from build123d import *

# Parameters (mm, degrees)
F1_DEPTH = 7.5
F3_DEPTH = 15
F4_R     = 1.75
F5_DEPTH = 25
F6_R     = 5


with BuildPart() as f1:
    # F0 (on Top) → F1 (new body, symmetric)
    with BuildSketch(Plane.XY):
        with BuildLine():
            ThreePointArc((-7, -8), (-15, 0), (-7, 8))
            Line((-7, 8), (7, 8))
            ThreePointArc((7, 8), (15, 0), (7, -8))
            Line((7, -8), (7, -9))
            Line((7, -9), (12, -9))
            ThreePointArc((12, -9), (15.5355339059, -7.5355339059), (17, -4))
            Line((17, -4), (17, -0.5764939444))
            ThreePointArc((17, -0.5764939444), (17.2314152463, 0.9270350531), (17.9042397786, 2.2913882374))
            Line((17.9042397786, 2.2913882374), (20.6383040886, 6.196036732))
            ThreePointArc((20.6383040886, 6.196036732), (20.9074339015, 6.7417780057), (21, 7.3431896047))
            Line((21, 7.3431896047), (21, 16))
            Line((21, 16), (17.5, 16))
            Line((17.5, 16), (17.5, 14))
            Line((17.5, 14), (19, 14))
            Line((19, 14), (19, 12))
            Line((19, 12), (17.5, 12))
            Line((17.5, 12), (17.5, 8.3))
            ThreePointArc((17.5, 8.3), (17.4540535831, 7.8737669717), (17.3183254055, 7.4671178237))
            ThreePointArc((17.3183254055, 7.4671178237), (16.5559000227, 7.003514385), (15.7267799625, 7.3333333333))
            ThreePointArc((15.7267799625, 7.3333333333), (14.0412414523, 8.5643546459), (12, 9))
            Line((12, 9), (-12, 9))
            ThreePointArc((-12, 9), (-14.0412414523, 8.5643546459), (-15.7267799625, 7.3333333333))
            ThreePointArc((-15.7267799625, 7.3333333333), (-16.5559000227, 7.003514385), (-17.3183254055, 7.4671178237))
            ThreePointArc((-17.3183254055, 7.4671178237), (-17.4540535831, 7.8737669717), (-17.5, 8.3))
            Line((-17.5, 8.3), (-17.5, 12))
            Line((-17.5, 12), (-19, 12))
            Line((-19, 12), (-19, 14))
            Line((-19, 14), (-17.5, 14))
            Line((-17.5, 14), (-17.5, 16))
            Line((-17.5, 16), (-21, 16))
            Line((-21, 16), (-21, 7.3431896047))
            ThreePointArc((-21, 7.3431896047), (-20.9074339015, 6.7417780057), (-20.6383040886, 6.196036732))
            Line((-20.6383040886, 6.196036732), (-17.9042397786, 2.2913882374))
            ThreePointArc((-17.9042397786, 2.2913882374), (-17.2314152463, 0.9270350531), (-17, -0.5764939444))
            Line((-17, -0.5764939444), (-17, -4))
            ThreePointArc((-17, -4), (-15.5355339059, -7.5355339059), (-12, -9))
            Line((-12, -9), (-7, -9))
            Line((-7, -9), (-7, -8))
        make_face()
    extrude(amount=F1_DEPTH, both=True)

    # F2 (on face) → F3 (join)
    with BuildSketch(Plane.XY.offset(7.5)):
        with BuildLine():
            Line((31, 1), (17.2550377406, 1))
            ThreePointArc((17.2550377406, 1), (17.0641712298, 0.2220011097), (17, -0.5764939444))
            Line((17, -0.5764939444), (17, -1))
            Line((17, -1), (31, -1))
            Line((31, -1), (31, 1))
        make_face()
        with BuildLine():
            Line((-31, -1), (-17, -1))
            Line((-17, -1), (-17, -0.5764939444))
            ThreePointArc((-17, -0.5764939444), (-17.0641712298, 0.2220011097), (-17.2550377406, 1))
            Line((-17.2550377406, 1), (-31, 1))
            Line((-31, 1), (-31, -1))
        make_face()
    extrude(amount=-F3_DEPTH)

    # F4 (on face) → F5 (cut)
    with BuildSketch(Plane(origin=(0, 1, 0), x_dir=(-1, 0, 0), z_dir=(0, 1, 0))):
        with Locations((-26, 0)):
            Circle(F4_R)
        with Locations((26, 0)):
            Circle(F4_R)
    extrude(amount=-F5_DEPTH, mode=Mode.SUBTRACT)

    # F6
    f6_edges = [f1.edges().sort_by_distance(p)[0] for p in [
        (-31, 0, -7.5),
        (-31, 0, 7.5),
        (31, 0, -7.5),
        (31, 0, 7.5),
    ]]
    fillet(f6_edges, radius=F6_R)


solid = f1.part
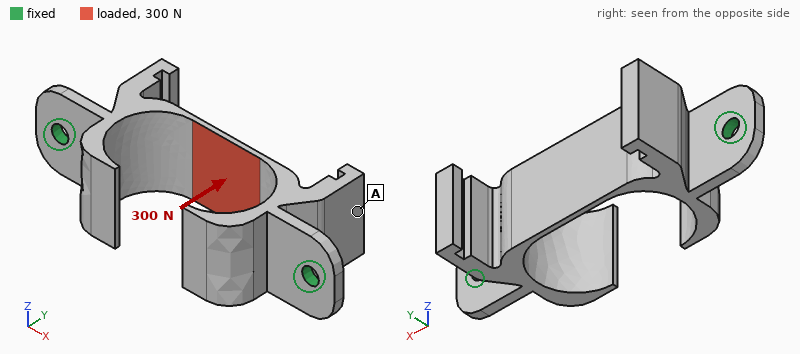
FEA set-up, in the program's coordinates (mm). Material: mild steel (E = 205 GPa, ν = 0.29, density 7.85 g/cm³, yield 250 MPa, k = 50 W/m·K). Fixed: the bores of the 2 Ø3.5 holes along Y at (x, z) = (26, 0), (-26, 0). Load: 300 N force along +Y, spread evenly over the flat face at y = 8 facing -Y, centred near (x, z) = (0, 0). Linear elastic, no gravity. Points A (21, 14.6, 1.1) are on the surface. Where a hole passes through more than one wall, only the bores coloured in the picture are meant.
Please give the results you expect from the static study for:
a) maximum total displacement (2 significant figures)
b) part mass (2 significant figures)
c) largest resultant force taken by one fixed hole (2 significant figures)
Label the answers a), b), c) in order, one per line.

a) 39 µm
b) 34 g
c) 310 N
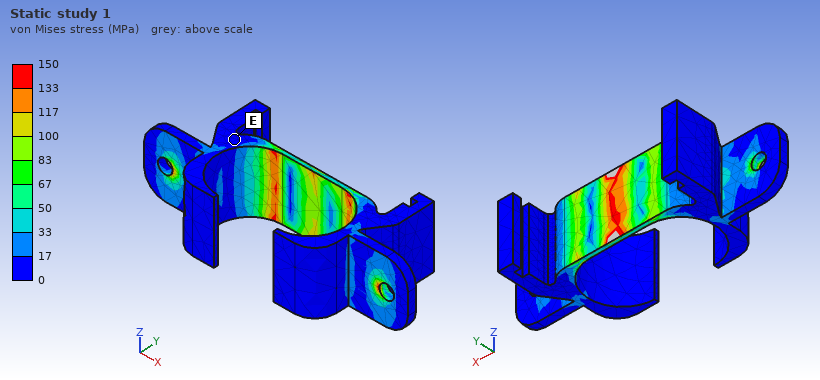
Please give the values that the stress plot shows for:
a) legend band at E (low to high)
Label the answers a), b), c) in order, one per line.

a) 0 to 17 MPa
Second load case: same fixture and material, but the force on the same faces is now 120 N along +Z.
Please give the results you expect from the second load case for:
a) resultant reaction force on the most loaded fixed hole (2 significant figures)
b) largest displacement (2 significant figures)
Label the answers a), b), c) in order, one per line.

a) 60 N
b) 18 µm
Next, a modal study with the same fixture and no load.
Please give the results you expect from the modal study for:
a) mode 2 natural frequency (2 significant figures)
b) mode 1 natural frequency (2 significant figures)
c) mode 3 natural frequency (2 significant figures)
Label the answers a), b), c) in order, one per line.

a) 3300 Hz
b) 3300 Hz
c) 4500 Hz
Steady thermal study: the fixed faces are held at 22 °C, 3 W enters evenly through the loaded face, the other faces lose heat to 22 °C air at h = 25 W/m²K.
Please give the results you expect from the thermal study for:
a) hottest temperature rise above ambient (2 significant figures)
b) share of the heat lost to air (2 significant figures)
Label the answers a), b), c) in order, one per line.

a) 25 K
b) 29 %
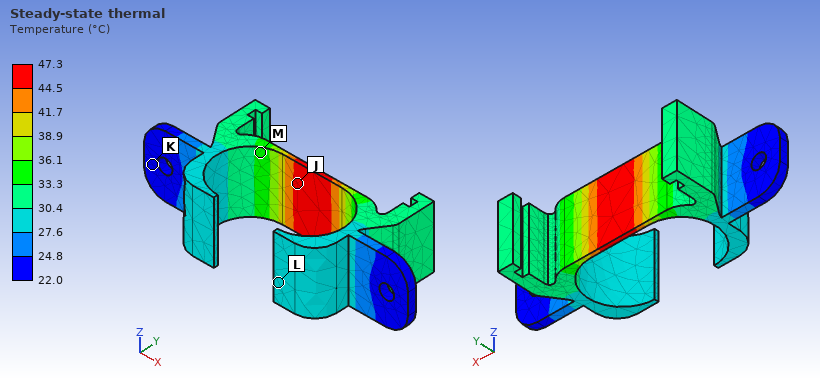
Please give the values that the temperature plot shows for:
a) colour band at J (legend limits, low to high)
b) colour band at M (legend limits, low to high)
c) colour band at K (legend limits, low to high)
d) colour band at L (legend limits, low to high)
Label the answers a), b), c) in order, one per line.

a) 44.5 to 47.3 °C
b) 33.3 to 36.1 °C
c) 22.0 to 24.8 °C
d) 27.6 to 30.4 °C
